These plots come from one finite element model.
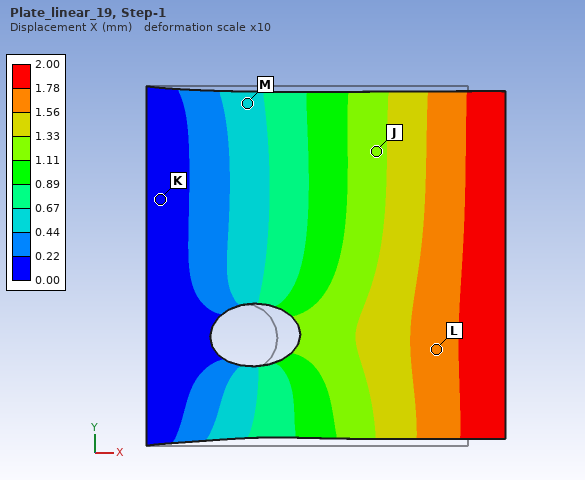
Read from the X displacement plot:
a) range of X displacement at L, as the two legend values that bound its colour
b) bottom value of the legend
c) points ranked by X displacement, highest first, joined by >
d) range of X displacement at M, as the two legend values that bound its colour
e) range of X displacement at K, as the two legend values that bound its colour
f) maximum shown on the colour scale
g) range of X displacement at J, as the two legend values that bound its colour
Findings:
1.56 to 1.78 mm
0.00 mm
L > J > M > K
0.44 to 0.67 mm
0.00 to 0.22 mm
2.00 mm
1.11 to 1.33 mm
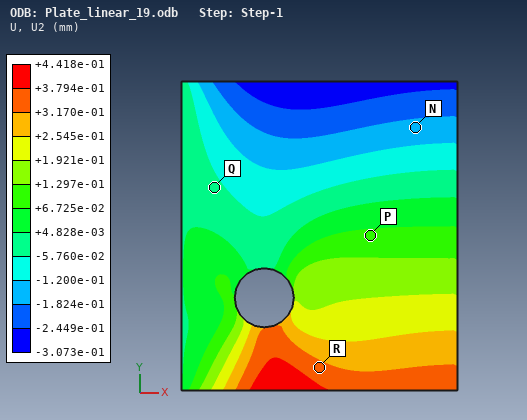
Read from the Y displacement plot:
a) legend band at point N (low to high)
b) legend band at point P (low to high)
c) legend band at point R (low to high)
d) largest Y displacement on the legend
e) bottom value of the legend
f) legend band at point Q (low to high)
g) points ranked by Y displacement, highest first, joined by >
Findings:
-1.824e-01 to -1.200e-01 mm
+6.725e-02 to +1.297e-01 mm
+3.170e-01 to +3.794e-01 mm
+4.418e-01 mm
-3.073e-01 mm
-5.760e-02 to +4.828e-03 mm
R > P > Q > N
